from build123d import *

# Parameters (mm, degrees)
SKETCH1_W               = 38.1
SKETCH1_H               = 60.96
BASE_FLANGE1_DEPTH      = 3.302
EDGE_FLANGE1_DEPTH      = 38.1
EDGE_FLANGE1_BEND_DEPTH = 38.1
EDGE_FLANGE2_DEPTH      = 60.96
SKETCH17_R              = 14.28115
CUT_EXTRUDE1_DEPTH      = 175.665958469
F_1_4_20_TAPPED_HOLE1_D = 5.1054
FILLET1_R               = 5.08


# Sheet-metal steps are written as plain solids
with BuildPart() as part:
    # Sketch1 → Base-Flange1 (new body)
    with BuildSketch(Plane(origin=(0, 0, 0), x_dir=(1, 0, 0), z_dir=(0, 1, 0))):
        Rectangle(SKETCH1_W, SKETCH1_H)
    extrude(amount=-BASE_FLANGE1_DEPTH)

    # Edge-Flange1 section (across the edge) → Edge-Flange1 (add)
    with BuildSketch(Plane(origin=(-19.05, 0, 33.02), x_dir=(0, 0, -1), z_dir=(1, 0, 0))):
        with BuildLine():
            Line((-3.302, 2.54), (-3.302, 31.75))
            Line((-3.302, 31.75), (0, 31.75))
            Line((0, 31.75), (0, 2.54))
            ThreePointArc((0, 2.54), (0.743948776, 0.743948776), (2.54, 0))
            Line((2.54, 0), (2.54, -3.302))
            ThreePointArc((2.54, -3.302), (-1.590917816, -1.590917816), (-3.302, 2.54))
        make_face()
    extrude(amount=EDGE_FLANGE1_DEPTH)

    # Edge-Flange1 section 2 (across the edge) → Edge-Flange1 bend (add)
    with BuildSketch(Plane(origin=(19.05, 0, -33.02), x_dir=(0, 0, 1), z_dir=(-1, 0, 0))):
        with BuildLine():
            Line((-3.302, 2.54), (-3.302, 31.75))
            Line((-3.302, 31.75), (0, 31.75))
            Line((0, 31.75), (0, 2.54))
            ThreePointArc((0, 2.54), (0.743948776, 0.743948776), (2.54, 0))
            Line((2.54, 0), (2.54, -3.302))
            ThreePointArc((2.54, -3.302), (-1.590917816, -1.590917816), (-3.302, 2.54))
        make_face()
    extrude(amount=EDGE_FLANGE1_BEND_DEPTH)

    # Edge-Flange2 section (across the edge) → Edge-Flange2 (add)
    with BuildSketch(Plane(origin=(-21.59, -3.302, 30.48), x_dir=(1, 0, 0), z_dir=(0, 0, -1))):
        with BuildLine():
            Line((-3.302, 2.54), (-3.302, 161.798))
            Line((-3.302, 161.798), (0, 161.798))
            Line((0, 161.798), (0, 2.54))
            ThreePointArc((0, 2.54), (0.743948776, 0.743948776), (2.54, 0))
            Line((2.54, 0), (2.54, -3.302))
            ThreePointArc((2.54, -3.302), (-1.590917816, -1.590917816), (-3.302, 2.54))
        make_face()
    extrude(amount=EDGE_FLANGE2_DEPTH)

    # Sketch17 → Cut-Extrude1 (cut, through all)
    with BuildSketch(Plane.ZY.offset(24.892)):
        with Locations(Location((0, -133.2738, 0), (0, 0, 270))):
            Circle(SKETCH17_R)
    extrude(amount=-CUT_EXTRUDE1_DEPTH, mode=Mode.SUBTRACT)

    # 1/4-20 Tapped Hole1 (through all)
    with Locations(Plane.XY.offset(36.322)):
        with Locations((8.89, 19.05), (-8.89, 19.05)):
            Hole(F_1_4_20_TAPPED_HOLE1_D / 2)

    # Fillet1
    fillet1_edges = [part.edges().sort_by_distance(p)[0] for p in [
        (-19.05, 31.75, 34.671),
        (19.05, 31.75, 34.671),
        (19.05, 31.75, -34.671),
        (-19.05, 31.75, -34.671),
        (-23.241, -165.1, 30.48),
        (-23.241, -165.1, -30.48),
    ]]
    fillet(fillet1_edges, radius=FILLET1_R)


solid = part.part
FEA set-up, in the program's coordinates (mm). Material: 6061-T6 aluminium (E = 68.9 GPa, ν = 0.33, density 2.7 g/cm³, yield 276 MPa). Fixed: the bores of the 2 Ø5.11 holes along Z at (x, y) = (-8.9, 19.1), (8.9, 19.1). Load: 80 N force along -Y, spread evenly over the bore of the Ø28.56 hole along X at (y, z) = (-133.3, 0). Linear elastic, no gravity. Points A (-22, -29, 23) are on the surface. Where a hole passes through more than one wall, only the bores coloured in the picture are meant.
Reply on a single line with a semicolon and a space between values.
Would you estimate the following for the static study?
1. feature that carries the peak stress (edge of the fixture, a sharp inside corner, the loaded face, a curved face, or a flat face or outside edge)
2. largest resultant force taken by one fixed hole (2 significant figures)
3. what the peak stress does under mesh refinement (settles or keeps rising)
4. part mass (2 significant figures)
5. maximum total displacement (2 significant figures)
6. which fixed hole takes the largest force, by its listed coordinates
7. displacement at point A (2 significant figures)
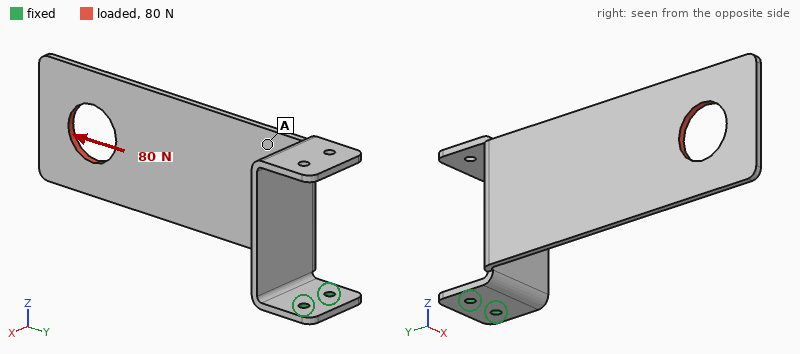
a sharp inside corner; 130 N; keeps rising; 130 g; 2.1 mm; (-8.9, 19.1); 0.77 mm
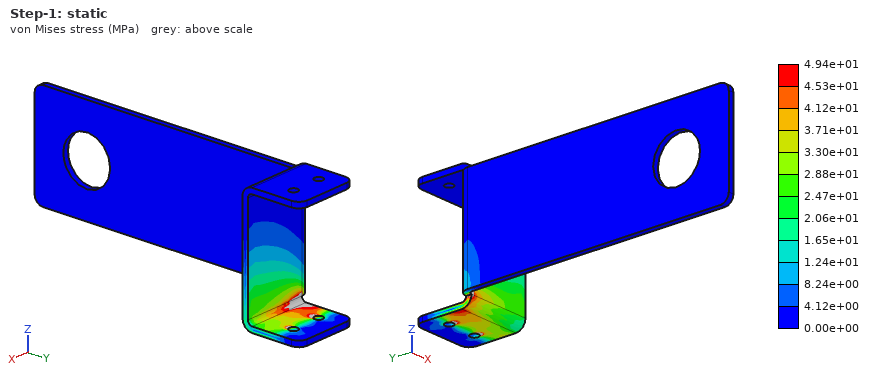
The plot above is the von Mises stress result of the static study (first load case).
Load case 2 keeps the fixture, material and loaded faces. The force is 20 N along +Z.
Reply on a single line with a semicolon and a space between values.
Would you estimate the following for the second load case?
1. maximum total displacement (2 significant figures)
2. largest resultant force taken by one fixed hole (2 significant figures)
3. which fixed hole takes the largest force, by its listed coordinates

2.2 mm; 35 N; (-8.9, 19.1)
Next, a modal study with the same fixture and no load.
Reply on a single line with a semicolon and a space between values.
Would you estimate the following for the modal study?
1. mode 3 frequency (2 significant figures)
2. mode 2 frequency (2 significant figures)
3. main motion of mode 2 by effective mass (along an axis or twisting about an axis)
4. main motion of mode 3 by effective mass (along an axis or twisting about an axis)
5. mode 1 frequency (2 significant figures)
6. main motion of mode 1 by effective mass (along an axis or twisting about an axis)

400 Hz; 91 Hz; along X; along X; 74 Hz; along Z
